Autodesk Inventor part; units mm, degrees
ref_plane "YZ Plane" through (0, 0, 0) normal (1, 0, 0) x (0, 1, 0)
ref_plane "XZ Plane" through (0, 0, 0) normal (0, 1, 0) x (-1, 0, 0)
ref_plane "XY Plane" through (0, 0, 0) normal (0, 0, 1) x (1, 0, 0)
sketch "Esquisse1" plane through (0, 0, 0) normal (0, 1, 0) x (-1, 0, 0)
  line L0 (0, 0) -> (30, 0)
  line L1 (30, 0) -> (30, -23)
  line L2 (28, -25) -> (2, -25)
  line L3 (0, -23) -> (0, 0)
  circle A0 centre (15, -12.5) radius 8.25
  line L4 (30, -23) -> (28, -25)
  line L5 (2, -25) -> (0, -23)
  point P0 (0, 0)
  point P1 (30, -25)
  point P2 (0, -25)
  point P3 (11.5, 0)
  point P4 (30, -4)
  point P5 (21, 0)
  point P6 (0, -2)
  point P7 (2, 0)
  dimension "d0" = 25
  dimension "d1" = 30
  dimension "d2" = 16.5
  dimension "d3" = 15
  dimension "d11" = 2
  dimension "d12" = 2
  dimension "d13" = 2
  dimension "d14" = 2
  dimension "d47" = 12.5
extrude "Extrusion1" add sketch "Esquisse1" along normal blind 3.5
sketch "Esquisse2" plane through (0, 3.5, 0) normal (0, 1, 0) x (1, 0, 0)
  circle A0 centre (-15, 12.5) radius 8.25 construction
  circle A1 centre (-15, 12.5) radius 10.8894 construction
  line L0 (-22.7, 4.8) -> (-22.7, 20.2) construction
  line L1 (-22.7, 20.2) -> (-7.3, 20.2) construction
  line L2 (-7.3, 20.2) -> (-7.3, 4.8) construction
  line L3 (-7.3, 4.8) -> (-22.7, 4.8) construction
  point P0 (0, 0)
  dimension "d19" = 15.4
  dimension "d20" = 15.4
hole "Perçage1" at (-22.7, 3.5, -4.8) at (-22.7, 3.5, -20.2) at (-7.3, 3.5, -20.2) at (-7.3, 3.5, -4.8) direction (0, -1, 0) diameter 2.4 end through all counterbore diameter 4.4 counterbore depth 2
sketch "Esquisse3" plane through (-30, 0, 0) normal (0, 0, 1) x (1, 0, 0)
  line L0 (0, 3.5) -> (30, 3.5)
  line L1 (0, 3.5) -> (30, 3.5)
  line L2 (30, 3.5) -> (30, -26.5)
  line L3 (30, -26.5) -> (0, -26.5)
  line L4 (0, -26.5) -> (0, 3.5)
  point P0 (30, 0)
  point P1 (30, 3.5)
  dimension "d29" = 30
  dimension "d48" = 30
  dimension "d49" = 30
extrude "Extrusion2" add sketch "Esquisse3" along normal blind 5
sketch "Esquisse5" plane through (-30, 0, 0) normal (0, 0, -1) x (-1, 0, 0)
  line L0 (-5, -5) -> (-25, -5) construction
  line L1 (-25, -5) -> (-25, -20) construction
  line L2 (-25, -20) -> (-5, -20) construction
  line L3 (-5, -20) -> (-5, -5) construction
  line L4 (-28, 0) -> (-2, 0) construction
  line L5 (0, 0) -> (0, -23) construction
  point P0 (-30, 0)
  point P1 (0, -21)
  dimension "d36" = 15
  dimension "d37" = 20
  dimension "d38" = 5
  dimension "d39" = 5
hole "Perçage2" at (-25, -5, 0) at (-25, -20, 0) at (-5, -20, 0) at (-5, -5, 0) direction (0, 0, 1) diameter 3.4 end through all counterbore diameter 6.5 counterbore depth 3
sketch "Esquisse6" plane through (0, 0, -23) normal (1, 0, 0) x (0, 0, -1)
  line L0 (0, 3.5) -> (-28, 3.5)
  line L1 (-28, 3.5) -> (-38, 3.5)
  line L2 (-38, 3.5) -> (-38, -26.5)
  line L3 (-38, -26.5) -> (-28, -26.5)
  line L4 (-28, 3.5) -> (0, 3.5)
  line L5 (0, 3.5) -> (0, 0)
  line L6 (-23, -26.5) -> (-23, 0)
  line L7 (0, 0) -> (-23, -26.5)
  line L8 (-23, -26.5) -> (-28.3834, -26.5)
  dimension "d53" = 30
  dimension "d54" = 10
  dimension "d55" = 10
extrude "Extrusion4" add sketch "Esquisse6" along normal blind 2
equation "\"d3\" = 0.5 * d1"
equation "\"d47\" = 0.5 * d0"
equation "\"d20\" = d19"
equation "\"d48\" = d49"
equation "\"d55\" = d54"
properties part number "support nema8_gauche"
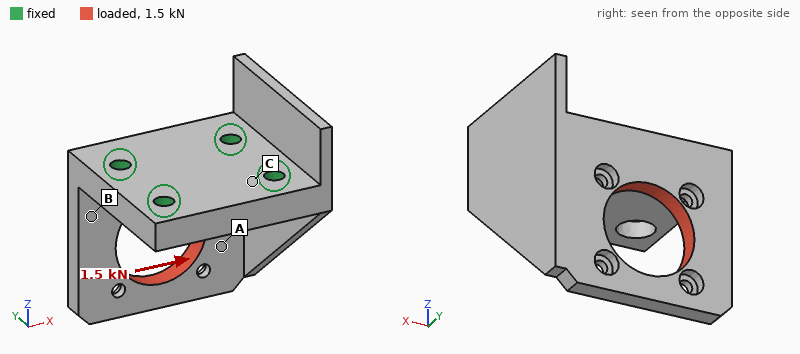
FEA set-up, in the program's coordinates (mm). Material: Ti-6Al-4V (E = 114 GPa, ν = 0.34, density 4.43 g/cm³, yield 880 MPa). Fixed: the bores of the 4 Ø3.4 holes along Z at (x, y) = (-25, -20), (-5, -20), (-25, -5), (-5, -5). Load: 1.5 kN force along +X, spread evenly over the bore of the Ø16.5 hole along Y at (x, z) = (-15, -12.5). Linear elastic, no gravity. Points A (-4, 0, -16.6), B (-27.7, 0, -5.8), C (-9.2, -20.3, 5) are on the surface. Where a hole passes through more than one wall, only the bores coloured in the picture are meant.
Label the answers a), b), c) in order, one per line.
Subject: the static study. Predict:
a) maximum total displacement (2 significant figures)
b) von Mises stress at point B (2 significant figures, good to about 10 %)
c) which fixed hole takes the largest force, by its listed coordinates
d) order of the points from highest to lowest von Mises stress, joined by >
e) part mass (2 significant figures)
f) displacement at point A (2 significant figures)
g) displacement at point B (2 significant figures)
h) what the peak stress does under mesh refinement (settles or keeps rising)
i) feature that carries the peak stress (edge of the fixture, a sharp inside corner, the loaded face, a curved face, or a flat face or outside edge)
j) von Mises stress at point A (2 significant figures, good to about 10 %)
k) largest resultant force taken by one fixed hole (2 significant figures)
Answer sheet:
a) 67 µm
b) 63 MPa
c) (-25, -5)
d) B > A > C
e) 33 g
f) 47 µm
g) 28 µm
h) keeps rising
i) edge of the fixture
j) 38 MPa
k) 1.5 kN
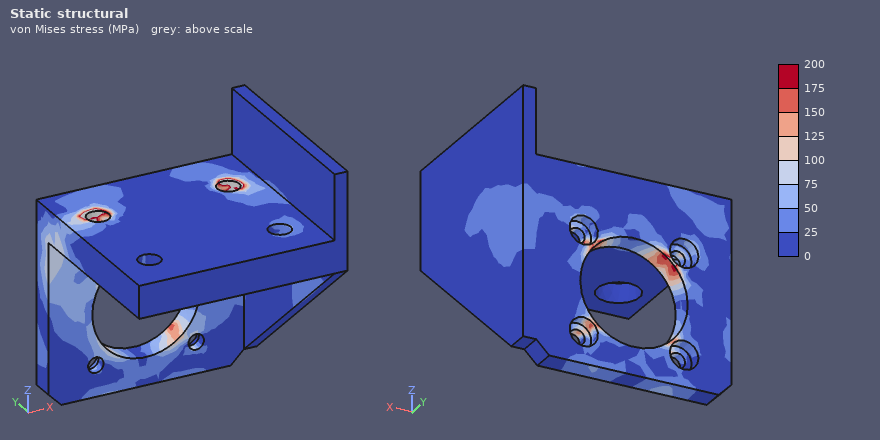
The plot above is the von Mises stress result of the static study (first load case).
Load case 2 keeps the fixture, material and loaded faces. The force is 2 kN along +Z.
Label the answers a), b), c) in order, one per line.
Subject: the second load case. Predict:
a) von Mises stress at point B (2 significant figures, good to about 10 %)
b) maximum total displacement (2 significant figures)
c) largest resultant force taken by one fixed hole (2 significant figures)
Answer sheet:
a) 40 MPa
b) 68 µm
c) 1.4 kN
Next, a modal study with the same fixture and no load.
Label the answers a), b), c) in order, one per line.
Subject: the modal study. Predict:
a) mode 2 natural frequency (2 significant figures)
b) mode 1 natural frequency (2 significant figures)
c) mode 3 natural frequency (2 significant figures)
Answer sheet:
a) 8100 Hz
b) 4400 Hz
c) 11 kHz
